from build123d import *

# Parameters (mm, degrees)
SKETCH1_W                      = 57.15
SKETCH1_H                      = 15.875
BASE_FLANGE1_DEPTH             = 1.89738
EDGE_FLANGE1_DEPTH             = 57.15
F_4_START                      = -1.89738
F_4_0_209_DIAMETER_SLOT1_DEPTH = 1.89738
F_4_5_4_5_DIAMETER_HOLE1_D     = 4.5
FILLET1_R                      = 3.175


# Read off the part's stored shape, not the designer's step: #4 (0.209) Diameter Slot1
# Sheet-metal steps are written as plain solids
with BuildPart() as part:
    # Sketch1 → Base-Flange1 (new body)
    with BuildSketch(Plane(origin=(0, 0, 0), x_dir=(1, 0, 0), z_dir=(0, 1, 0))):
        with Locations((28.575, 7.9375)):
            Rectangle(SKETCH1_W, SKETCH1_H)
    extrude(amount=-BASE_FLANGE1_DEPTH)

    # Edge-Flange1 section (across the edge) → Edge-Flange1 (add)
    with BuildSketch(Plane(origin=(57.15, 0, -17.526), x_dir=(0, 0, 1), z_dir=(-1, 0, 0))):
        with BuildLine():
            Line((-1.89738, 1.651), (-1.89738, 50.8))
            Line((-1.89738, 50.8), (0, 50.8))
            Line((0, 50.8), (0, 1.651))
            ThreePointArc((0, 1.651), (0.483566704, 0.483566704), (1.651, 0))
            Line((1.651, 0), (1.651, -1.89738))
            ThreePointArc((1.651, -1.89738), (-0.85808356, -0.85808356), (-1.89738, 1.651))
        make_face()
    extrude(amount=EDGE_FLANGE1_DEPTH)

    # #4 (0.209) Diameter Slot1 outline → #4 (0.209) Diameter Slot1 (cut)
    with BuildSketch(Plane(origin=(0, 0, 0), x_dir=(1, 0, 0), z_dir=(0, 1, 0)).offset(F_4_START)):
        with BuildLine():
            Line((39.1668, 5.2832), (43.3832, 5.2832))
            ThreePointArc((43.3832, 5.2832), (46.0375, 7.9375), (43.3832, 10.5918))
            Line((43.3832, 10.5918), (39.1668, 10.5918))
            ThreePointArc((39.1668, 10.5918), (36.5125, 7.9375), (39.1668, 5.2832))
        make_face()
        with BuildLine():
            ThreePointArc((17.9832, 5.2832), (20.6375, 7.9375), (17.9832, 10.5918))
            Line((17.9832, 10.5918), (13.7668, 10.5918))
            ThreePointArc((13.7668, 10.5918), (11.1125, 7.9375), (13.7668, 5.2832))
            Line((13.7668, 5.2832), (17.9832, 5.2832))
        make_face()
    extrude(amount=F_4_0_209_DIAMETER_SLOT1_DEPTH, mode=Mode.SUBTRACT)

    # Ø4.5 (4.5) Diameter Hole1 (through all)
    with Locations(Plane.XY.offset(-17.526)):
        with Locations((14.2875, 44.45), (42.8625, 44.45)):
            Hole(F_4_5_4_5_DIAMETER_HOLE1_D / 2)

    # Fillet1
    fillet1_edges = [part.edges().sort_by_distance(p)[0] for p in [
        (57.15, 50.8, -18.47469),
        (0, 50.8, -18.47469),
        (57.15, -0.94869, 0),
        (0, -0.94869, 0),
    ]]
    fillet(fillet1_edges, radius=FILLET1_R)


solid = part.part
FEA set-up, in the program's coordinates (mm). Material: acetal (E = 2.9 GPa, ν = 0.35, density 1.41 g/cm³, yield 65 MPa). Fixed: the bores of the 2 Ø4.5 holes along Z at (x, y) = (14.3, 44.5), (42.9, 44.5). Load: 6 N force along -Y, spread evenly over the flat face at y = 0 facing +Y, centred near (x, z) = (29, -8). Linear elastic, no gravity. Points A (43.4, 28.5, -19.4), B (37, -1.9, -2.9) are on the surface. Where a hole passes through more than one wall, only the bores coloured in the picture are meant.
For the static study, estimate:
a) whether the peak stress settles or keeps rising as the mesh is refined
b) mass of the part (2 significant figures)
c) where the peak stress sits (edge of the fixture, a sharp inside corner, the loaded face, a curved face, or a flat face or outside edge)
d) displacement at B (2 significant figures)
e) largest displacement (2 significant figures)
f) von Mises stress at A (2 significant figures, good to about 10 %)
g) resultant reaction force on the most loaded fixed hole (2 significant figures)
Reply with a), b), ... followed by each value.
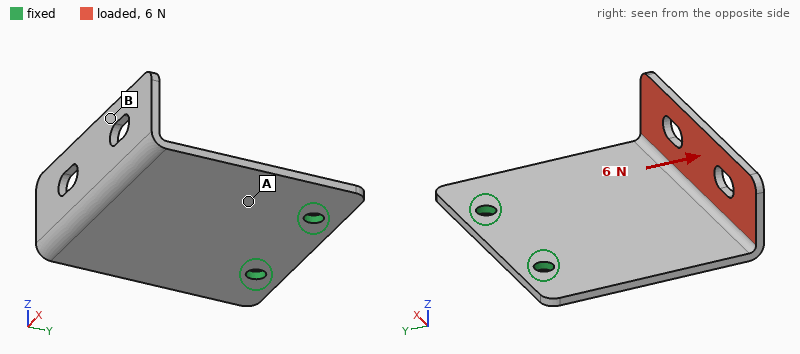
a) keeps rising
b) 10 g
c) edge of the fixture
d) 0.83 mm
e) 0.89 mm
f) 1.6 MPa
g) 3.0 N
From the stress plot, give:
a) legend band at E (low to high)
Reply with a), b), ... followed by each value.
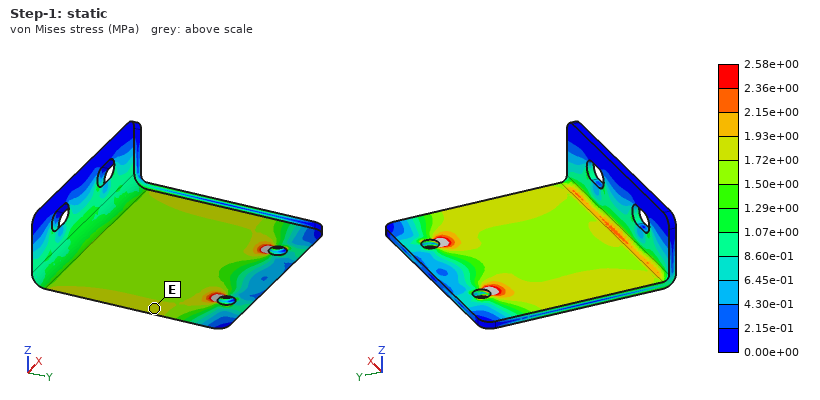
a) 1.72e+00 to 1.93e+00 MPa
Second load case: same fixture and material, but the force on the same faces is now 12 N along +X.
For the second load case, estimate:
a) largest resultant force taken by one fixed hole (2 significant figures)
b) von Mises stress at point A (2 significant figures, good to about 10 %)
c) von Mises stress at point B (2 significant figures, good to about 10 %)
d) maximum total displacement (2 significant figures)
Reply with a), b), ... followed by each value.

a) 18 N
b) 2.1 MPa
c) 1.2 MPa
d) 0.88 mm
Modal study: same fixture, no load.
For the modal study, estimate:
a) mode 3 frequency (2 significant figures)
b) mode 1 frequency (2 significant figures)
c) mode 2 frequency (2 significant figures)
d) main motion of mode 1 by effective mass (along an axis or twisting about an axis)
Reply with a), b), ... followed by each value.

a) 650 Hz
b) 140 Hz
c) 280 Hz
d) along Z
